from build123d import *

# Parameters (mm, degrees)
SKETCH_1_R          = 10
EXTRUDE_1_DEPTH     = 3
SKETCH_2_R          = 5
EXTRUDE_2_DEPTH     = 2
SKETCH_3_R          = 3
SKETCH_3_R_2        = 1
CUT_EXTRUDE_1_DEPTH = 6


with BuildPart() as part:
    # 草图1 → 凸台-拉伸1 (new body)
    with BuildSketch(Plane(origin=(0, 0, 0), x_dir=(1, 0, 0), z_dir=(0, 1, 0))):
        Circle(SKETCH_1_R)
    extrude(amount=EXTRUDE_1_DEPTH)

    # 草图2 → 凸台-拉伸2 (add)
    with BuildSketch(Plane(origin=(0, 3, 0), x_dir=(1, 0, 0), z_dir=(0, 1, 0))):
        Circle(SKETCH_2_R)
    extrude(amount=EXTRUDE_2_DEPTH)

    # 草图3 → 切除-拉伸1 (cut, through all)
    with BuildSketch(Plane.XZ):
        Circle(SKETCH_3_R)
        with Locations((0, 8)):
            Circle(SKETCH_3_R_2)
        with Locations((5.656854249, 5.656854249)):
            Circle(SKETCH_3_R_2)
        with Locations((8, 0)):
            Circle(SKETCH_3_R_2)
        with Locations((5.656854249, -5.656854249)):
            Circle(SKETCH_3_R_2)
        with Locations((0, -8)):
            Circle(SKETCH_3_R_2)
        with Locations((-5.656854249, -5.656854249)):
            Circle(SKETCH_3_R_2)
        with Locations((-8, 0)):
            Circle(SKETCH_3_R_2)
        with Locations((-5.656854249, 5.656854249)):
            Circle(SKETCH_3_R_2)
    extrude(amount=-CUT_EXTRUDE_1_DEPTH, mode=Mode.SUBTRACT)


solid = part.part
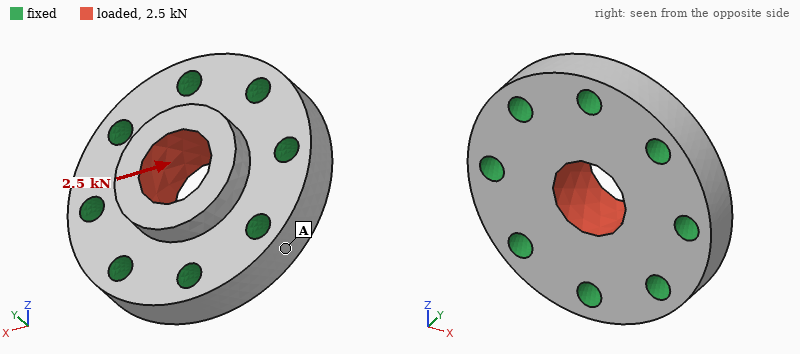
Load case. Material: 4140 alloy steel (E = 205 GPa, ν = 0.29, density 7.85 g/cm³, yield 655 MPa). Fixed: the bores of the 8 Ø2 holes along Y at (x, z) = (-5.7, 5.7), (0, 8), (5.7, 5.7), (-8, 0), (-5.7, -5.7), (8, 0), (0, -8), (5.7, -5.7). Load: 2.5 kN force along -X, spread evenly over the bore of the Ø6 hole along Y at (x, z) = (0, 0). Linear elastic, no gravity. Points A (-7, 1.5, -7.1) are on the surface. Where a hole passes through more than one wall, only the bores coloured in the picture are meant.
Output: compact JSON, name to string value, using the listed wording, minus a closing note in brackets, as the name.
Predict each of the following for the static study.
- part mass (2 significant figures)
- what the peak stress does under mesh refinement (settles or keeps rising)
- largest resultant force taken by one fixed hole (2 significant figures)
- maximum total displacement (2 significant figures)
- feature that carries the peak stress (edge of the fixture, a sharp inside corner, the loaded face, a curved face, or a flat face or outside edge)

{"part mass": "6.9 g", "what the peak stress does under mesh refinement": "keeps rising", "largest resultant force taken by one fixed hole": "510 N", "maximum total displacement": "2.0 µm", "feature that carries the peak stress": "a sharp inside corner"}
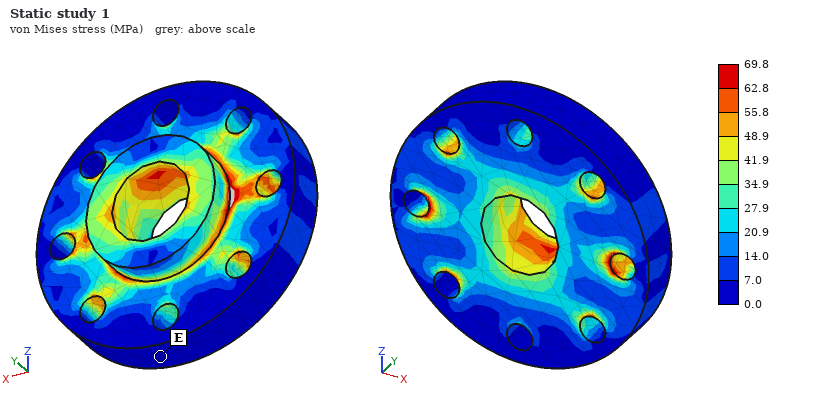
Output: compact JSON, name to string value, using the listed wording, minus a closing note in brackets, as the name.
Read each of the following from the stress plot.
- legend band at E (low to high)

{"legend band at E": "0.0 to 7.0 MPa"}
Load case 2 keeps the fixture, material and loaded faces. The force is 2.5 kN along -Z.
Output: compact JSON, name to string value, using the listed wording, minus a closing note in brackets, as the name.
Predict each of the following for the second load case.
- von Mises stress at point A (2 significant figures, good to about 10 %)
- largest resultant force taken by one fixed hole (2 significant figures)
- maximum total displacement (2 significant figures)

{"von Mises stress at point A": "5.7 MPa", "largest resultant force taken by one fixed hole": "500 N", "maximum total displacement": "1.9 µm"}
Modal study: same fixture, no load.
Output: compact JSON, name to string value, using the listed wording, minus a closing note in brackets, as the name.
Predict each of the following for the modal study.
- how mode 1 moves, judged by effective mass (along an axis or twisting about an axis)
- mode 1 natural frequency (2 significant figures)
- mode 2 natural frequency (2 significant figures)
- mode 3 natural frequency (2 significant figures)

{"how mode 1 moves, judged by effective mass": "along Y", "mode 1 natural frequency": "110 kHz", "mode 2 natural frequency": "140 kHz", "mode 3 natural frequency": "140 kHz"}
